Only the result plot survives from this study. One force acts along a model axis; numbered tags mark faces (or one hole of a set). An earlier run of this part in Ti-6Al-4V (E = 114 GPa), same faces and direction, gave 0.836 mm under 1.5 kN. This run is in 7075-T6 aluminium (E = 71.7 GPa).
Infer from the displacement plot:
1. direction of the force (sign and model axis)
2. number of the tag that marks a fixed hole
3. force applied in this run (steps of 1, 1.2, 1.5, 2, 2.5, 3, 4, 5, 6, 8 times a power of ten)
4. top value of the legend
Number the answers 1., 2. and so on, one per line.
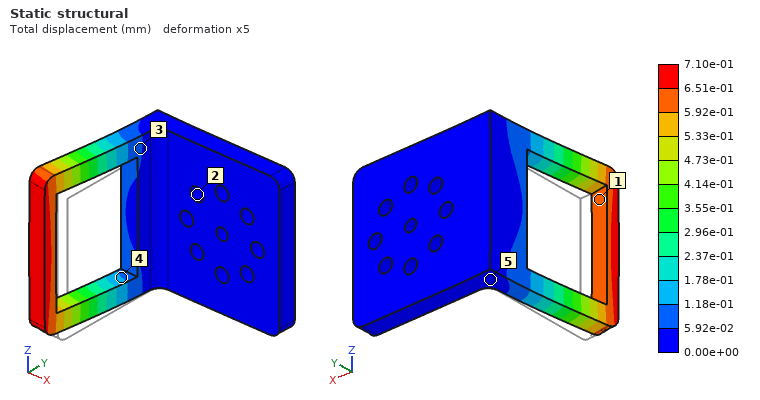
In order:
1. -X
2. 2
3. 800 N
4. 7.10e-01 mm
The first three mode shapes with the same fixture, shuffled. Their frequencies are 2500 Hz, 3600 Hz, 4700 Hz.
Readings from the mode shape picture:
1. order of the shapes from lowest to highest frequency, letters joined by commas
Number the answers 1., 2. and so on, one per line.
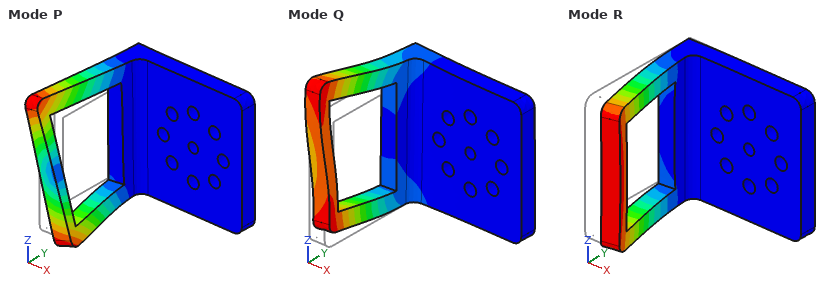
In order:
1. R, Q, P
